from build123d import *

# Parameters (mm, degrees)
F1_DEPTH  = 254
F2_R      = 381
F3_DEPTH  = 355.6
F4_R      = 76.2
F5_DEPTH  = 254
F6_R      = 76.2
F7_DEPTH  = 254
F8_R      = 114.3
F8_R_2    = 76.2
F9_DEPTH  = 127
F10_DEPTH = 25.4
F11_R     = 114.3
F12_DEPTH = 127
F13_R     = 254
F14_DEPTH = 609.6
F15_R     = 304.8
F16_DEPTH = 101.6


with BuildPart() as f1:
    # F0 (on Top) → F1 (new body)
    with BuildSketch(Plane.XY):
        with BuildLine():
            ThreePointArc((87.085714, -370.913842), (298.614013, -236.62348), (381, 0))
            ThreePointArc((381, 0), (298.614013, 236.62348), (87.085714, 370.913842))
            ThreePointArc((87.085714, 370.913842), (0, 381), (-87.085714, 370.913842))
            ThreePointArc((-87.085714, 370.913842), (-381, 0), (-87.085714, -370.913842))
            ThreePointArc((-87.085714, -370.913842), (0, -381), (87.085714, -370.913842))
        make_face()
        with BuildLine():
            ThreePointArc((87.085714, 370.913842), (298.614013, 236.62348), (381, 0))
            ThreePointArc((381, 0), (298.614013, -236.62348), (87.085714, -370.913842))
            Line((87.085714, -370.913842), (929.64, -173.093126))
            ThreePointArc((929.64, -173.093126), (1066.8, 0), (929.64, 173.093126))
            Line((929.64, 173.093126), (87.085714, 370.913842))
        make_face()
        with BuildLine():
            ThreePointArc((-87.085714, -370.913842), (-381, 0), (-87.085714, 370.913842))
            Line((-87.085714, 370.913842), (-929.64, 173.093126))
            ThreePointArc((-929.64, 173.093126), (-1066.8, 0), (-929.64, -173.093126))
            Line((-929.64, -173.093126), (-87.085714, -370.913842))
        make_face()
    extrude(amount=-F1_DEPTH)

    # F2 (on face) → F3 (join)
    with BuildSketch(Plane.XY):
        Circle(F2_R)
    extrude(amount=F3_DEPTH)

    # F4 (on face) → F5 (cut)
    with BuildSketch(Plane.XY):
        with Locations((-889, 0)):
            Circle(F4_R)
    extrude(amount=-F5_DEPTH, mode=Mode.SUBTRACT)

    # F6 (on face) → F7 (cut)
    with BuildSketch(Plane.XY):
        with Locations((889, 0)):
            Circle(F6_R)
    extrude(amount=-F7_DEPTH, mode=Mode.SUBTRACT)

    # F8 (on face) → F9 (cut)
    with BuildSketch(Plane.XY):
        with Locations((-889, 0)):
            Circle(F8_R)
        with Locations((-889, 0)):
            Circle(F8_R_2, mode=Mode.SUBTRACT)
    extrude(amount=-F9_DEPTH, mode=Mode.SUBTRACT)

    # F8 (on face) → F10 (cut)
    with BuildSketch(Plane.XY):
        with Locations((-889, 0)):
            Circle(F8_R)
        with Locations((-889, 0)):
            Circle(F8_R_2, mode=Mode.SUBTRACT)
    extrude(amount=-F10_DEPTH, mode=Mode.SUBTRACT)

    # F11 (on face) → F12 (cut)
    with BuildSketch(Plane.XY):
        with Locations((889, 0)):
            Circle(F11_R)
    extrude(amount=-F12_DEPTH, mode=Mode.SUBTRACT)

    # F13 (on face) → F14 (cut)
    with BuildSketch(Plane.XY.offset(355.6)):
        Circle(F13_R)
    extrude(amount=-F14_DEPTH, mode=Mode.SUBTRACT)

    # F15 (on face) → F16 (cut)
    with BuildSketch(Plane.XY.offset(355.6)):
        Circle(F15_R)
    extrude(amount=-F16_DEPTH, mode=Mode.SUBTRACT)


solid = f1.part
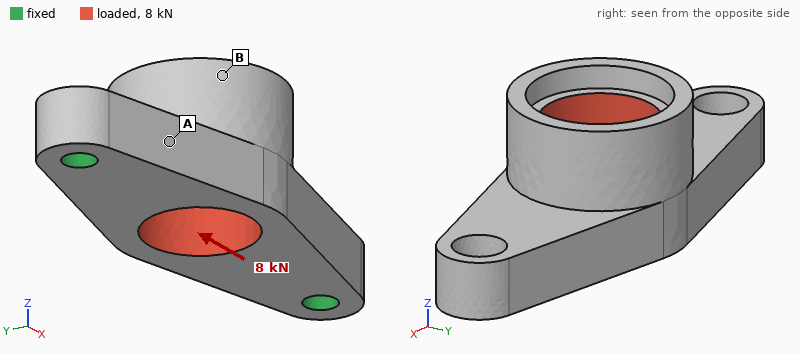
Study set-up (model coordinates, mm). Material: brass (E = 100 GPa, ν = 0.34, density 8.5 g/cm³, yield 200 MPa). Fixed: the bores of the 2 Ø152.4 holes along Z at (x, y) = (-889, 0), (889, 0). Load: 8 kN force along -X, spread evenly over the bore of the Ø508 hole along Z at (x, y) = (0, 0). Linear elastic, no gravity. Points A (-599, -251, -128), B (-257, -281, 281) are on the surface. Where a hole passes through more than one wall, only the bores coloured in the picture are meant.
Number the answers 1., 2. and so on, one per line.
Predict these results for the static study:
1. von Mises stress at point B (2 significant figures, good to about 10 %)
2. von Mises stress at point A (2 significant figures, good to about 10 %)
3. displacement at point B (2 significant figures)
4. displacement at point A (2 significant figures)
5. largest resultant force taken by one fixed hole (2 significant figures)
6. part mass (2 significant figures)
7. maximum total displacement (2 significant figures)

1. 0.012 MPa
2. 0.037 MPa
3. 0.52 µm
4. 0.19 µm
5. 4.1 kN
6. 2500 kg
7. 0.57 µm
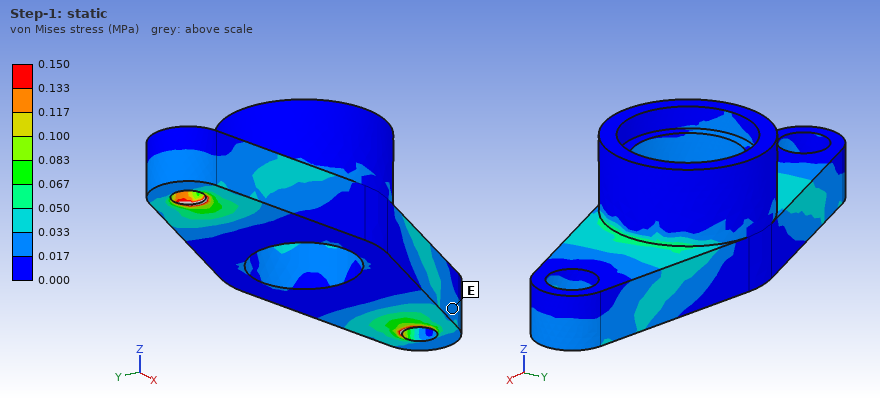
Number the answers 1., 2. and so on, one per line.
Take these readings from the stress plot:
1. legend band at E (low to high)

1. 0.017 to 0.033 MPa
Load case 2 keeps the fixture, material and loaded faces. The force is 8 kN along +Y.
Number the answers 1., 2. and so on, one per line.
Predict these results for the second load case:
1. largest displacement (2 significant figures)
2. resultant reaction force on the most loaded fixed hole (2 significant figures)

1. 6.8 µm
2. 4.0 kN
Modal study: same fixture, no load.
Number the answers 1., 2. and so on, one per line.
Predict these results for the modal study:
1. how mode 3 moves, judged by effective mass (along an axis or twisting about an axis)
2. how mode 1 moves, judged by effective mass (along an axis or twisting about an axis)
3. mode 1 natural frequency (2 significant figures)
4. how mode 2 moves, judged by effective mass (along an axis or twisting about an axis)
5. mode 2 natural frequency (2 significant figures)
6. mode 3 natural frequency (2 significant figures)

1. along Y
2. along Y
3. 140 Hz
4. along Z
5. 180 Hz
6. 330 Hz
